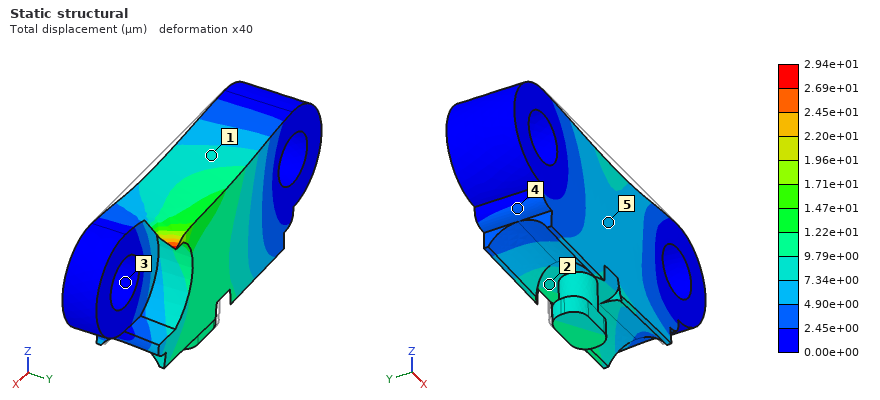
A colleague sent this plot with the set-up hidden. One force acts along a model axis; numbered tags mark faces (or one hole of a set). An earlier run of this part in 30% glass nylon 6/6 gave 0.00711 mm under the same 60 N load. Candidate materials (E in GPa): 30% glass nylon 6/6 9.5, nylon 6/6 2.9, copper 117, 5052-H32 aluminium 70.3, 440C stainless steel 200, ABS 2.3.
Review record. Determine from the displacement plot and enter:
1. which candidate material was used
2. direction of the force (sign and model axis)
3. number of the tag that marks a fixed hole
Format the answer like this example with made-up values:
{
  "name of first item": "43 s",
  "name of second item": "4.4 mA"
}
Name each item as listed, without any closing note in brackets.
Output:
{
  "which candidate material was used": "ABS",
  "direction of the force": "-Z",
  "number of the tag that marks a fixed hole": "3"
}
